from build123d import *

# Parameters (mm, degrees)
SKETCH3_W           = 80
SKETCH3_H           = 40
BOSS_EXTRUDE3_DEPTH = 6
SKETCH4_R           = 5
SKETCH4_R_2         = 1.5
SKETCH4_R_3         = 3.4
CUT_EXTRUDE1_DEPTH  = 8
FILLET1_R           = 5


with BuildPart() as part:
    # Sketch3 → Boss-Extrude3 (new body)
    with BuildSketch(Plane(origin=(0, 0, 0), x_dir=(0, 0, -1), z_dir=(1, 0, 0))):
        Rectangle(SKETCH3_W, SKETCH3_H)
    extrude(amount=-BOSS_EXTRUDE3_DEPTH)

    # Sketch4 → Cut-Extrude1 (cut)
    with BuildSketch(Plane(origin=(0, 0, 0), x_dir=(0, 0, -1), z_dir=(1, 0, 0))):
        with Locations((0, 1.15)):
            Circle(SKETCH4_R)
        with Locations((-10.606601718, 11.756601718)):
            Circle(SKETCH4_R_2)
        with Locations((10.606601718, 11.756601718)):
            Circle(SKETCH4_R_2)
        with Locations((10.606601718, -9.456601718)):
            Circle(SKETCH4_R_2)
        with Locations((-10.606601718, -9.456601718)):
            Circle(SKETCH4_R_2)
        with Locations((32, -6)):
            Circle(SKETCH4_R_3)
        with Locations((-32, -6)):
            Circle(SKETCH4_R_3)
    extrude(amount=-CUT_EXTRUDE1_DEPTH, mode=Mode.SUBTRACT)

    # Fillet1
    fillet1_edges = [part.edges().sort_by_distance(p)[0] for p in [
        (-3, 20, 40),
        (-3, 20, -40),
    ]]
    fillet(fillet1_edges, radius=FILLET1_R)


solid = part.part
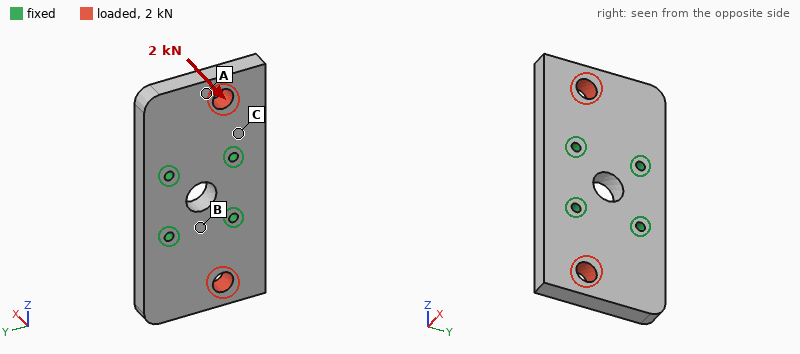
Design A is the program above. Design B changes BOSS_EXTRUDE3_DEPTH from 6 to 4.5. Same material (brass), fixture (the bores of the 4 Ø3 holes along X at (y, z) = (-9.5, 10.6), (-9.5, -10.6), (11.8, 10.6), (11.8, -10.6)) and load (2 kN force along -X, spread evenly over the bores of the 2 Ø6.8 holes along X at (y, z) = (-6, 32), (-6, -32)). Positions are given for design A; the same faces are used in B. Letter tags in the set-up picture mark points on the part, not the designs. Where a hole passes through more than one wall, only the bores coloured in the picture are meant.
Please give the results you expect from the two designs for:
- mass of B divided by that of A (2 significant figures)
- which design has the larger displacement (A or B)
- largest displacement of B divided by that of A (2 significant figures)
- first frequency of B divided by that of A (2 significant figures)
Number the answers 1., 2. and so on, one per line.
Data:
1. 0.75
2. B
3. 2.2
4. 0.78
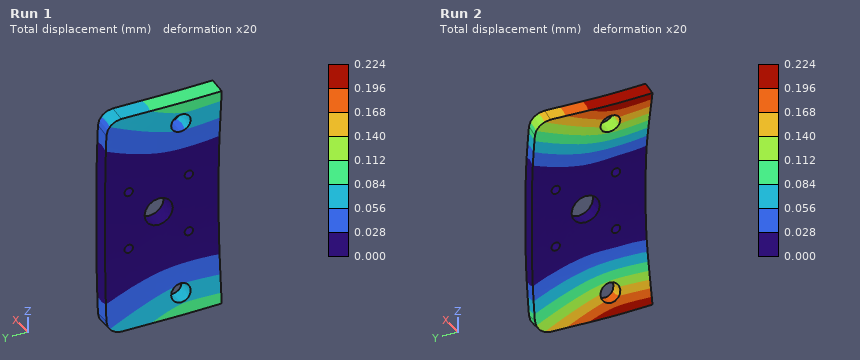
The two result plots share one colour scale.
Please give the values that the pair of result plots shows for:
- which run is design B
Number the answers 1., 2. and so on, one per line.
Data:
1. Run 2
